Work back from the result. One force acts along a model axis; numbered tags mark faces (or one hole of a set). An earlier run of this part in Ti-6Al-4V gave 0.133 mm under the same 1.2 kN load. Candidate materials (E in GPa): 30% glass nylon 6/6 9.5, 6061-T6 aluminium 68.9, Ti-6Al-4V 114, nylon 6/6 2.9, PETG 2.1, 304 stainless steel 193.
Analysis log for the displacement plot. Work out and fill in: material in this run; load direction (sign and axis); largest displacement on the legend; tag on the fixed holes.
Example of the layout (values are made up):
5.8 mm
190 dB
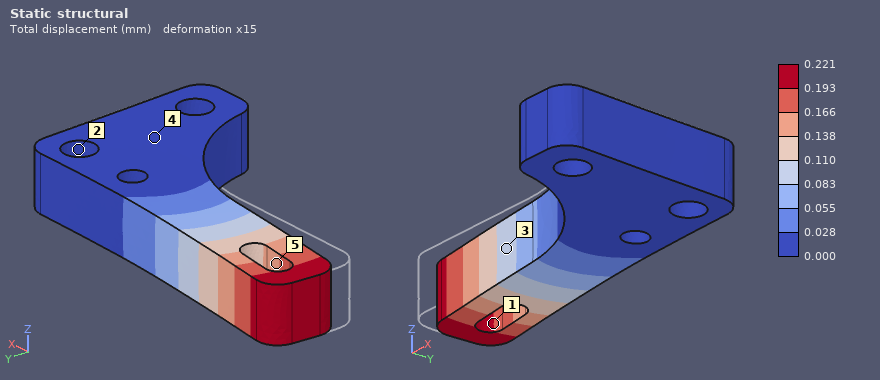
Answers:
6061-T6 aluminium
+Y
0.221 mm
2
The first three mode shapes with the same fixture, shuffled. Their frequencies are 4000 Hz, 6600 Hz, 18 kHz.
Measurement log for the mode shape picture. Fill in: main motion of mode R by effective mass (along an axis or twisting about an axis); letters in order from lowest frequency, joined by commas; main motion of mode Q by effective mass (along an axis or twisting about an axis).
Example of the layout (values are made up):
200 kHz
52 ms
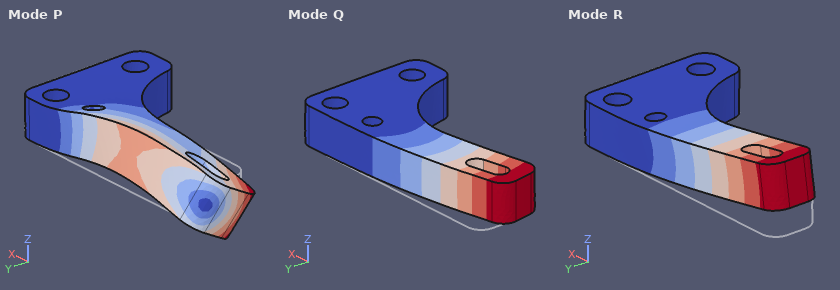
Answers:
along Z
R, Q, P
along Y
